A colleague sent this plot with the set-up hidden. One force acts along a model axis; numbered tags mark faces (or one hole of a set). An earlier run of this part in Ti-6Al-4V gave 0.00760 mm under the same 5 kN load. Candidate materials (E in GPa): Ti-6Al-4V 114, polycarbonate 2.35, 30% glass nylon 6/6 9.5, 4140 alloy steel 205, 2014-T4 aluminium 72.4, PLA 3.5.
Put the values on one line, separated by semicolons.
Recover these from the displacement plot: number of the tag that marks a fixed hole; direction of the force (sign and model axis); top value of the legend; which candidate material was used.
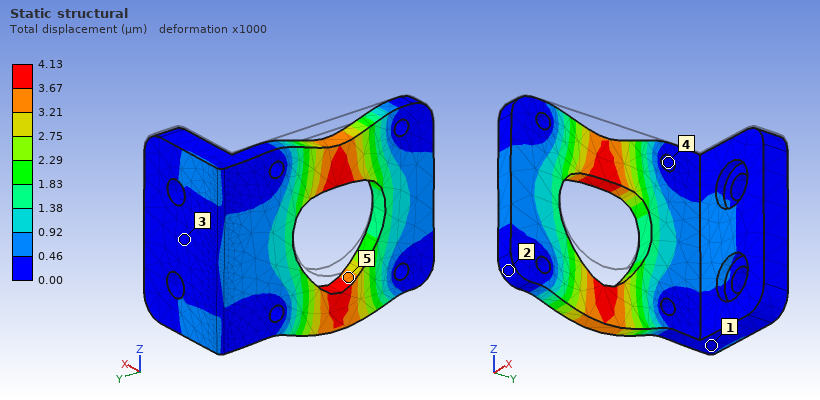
4; -Z; 4.13 µm; 4140 alloy steel
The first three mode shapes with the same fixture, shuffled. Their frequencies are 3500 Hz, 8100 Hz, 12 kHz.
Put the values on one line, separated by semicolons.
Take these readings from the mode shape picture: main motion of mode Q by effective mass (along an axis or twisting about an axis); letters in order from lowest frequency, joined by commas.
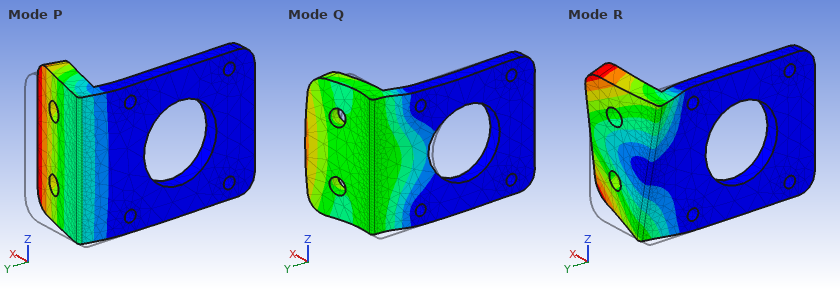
along X; P, R, Q
